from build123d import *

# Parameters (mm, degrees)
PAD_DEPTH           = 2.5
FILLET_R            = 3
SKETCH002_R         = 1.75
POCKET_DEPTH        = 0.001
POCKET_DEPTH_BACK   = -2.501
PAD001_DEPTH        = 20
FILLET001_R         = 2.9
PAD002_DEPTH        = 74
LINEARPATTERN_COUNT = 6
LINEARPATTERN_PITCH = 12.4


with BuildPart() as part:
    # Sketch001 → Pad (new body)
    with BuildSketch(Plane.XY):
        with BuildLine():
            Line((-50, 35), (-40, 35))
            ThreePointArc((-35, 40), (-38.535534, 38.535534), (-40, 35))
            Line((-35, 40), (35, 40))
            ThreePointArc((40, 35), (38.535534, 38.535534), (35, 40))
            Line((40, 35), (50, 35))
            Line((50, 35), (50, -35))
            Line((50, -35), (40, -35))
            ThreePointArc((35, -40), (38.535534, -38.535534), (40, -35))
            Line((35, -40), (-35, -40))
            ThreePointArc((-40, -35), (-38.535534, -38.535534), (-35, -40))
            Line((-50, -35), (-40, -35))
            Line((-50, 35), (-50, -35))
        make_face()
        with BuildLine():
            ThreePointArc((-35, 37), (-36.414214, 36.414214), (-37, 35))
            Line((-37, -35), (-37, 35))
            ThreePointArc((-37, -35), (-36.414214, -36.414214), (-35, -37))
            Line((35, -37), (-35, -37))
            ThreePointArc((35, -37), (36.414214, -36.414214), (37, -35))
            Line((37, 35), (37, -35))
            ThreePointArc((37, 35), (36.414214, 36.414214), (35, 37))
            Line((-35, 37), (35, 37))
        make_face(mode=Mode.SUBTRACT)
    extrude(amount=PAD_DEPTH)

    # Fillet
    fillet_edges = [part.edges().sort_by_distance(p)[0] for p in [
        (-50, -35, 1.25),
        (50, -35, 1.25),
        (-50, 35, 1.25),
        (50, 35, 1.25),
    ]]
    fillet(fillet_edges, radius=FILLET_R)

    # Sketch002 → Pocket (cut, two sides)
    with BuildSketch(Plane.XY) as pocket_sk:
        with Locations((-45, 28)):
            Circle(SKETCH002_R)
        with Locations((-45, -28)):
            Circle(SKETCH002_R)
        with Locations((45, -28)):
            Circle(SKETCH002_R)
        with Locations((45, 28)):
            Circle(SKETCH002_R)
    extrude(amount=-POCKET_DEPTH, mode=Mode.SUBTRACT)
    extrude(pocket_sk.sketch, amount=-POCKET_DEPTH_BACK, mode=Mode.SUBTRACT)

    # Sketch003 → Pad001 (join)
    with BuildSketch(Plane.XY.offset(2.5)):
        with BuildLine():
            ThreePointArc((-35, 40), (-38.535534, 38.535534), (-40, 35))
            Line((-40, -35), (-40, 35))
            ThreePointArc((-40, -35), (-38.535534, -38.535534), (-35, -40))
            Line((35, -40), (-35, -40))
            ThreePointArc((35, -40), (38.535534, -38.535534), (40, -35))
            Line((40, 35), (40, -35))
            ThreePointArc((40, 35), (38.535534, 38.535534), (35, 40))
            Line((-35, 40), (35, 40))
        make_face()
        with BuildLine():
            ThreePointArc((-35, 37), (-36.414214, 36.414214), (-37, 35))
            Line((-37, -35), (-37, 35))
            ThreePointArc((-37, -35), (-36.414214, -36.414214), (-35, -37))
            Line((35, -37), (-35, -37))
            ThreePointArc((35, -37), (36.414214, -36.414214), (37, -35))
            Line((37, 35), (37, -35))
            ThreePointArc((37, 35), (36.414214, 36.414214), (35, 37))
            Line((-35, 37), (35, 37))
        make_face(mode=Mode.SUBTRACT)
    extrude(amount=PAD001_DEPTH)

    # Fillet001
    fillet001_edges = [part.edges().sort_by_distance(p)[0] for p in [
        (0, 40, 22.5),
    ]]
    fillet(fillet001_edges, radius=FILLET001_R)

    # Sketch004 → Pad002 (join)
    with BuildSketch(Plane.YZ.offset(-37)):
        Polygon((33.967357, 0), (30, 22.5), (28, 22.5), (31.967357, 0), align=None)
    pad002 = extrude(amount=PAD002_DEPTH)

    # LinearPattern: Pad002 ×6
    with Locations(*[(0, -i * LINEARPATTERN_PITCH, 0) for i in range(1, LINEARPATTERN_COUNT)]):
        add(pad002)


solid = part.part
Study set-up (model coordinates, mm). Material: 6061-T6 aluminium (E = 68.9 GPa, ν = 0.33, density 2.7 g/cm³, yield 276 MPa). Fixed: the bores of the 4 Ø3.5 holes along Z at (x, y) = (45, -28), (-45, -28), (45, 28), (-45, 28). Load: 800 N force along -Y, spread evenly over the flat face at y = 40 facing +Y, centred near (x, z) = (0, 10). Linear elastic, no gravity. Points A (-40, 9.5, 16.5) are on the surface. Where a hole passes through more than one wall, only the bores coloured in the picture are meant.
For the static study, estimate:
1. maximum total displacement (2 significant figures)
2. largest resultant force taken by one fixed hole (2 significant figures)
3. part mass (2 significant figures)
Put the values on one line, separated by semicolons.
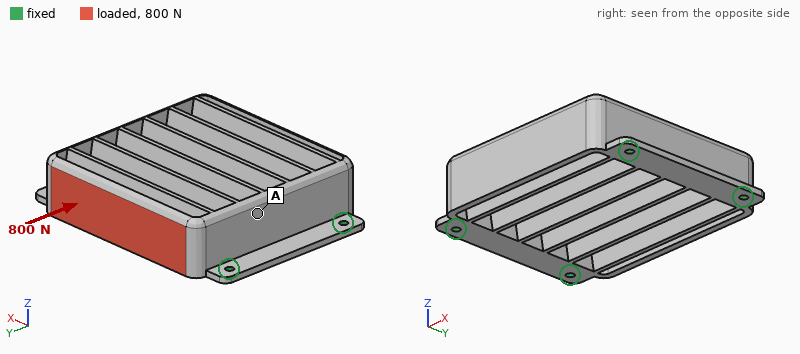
0.37 mm; 350 N; 120 g
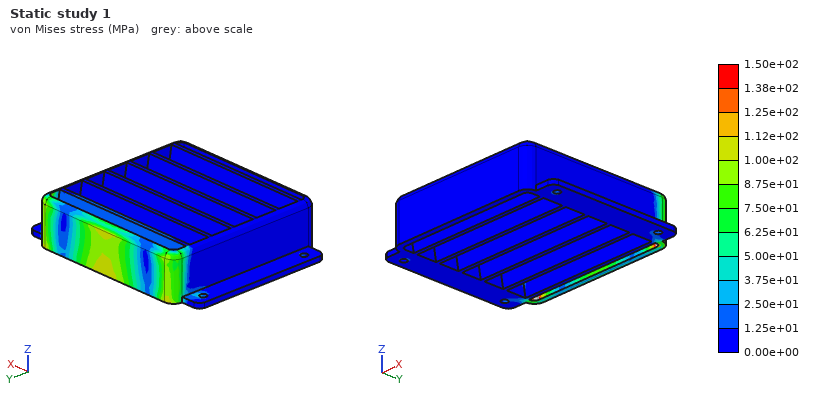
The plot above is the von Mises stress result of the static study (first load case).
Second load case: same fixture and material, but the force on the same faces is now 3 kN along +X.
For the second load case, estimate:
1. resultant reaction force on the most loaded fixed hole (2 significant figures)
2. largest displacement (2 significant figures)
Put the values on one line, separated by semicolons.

1.7 kN; 0.15 mm
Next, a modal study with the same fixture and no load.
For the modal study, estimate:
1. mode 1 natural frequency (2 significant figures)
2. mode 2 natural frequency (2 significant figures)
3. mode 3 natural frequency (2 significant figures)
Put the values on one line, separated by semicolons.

1800 Hz; 1800 Hz; 1800 Hz
